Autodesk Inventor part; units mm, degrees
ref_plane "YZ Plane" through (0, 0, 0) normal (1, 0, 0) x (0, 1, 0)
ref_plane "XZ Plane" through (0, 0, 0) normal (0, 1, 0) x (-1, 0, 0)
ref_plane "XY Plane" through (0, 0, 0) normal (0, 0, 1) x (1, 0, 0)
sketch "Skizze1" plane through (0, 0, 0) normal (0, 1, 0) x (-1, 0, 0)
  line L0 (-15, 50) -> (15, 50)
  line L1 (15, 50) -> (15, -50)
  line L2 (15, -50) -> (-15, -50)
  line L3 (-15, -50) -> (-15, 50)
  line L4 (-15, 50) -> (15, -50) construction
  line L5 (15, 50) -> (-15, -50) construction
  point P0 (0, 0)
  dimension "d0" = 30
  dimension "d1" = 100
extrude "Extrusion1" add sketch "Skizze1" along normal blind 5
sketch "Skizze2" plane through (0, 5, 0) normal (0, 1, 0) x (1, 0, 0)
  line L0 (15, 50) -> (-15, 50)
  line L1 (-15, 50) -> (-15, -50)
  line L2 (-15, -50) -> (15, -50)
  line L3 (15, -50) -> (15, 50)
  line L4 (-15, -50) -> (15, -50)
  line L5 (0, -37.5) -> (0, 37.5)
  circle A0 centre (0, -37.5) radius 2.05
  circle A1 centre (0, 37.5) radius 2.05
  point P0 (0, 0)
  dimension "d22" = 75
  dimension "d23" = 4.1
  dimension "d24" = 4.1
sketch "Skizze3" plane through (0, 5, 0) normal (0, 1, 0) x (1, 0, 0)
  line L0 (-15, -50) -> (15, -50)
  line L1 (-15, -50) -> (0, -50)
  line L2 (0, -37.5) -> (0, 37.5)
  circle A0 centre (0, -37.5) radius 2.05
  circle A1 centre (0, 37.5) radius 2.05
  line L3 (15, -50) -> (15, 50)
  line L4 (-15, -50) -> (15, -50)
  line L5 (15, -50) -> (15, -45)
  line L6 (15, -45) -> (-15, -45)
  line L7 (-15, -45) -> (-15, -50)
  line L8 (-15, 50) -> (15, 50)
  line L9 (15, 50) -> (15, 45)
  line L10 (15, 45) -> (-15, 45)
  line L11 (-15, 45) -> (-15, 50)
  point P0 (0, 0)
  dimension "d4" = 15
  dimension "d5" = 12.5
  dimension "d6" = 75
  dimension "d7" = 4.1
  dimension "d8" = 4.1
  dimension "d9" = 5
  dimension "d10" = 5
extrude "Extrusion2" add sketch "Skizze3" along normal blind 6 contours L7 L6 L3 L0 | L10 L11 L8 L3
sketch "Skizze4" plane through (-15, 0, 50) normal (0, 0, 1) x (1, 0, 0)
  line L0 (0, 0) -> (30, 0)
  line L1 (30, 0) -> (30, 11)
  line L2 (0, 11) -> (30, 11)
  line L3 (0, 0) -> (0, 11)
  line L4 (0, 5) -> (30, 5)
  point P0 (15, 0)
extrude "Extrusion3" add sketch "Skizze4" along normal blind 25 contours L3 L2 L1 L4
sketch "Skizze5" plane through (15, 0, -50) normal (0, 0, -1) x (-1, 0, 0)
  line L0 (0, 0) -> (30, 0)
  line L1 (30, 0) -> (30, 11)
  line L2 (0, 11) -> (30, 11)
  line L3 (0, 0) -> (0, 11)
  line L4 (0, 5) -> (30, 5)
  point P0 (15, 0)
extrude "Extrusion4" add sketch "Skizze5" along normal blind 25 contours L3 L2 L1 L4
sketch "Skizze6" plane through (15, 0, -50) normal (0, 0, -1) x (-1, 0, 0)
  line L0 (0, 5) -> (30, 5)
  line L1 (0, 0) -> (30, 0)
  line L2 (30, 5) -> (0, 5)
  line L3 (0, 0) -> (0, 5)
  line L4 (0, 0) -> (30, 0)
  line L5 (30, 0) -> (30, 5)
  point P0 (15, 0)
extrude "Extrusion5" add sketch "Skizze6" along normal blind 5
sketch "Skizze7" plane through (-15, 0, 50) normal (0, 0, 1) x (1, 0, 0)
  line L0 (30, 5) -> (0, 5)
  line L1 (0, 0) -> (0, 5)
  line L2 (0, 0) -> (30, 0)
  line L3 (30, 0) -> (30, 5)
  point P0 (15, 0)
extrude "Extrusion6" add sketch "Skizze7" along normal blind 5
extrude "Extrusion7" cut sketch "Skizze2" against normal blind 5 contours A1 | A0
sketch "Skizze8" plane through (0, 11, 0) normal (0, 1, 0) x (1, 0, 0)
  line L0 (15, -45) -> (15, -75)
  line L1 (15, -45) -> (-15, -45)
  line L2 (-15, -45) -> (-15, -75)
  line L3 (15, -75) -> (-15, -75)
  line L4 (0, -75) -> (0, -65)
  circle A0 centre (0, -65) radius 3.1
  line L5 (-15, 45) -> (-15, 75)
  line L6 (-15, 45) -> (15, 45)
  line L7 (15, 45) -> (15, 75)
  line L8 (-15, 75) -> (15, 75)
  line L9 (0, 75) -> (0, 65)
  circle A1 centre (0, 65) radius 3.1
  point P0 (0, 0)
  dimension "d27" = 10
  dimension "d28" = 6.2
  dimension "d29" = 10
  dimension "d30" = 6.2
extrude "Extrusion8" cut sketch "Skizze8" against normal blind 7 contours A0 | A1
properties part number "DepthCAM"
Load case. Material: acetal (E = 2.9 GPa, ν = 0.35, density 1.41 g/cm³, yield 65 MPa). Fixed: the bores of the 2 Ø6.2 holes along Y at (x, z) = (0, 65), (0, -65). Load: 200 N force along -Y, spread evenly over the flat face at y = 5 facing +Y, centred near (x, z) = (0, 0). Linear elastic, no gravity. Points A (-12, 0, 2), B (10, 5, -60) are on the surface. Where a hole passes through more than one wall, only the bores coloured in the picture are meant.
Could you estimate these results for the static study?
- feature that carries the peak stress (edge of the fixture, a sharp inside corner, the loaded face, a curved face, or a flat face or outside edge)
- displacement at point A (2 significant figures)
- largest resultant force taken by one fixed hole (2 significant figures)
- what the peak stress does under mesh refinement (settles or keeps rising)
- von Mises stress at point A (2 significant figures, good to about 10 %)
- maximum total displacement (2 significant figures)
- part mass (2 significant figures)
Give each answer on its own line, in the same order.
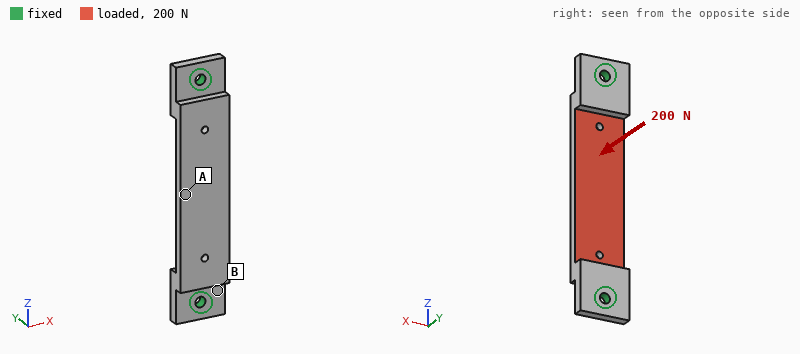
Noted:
edge of the fixture
0.83 mm
320 N
keeps rising
9.9 MPa
0.85 mm
38 g
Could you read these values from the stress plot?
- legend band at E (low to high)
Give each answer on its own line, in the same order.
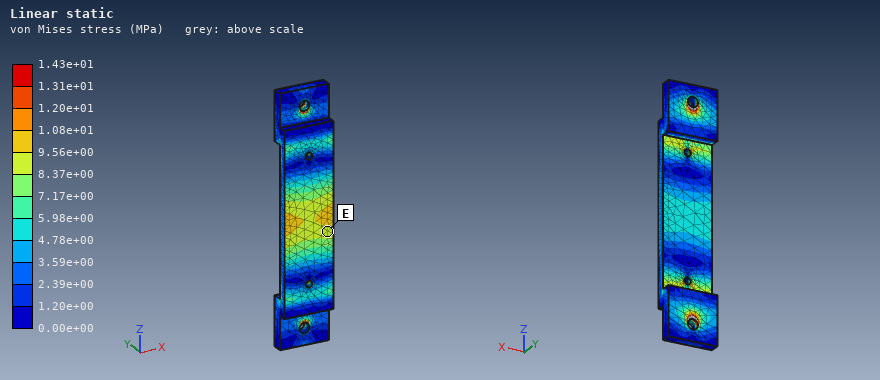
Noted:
8.37e+00 to 9.56e+00 MPa
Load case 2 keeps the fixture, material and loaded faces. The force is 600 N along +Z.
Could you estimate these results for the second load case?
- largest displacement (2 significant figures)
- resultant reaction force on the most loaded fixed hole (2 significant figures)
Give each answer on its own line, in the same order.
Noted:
0.18 mm
300 N
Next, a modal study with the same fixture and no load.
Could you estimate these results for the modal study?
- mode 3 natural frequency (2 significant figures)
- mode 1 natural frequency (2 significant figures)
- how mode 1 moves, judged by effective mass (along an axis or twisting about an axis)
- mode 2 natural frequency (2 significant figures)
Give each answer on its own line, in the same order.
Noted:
1300 Hz
640 Hz
along Y
1200 Hz
